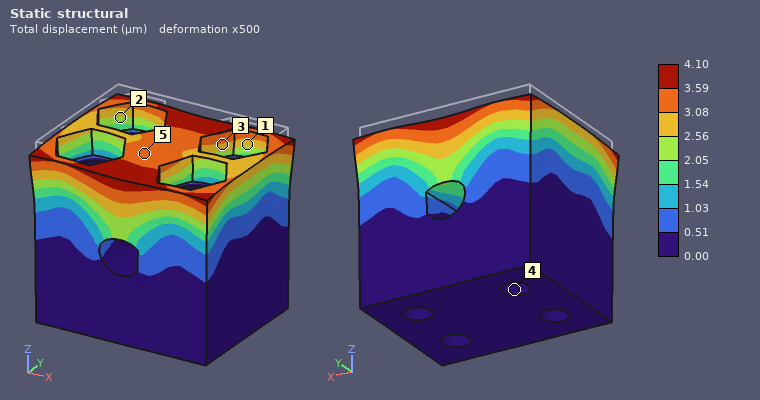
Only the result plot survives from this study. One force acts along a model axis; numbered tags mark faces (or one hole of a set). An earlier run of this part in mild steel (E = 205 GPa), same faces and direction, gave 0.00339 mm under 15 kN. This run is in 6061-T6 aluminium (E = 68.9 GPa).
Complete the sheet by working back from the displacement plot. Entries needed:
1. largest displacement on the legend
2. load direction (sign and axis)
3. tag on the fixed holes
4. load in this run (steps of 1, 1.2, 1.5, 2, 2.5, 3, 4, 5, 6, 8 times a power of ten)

4.10 µm
-Z
4
6 kN
